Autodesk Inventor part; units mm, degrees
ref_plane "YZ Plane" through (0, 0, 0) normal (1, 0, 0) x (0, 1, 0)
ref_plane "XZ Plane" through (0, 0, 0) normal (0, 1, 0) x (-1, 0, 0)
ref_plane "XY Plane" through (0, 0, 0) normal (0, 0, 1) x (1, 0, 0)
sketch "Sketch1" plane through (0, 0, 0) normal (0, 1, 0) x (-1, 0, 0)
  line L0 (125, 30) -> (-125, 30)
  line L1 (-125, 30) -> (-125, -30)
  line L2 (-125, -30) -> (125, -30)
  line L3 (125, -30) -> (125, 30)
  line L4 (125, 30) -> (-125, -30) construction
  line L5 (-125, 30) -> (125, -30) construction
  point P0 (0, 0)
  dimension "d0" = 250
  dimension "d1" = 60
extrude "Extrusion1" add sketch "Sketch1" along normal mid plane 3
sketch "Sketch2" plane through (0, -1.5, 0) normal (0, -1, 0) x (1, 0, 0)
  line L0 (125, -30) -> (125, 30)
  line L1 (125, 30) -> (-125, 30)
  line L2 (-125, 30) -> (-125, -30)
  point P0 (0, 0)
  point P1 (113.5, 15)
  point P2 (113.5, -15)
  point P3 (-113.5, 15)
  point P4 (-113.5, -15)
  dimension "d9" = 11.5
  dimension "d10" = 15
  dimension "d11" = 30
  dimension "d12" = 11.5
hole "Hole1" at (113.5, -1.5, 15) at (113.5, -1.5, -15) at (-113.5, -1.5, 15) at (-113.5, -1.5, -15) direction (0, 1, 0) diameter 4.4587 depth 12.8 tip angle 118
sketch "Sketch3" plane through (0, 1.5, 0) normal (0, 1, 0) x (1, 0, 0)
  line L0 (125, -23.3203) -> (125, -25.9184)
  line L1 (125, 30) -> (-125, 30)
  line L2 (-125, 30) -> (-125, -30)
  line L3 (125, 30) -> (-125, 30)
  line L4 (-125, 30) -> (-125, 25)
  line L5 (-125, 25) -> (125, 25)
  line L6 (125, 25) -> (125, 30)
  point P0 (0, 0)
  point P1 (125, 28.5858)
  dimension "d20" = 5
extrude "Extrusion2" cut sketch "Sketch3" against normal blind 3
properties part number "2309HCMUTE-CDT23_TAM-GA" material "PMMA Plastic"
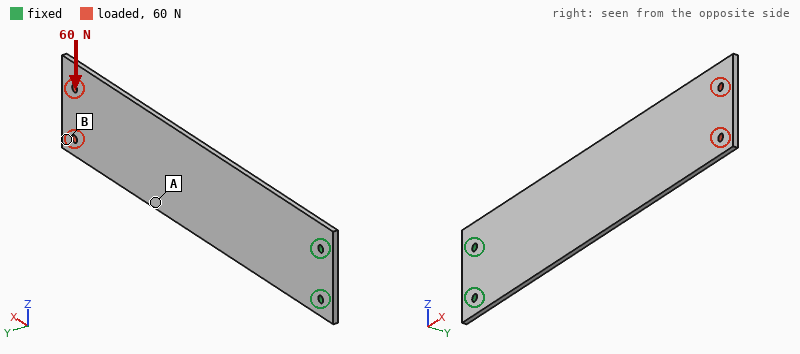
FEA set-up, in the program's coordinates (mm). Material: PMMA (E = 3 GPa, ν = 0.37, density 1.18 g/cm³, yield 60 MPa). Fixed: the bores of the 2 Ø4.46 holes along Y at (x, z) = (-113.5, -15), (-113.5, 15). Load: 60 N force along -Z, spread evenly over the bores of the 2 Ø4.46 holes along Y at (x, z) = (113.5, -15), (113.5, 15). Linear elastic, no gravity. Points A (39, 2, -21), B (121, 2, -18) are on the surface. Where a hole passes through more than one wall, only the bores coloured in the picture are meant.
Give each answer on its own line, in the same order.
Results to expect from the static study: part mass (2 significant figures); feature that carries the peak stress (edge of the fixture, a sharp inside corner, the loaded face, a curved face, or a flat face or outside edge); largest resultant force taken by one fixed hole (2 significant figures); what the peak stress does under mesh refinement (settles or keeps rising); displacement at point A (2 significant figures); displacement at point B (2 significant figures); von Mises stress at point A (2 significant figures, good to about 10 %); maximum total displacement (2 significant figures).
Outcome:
48 g
edge of the fixture
430 N
keeps rising
1.3 mm
2.4 mm
2.6 MPa
2.4 mm
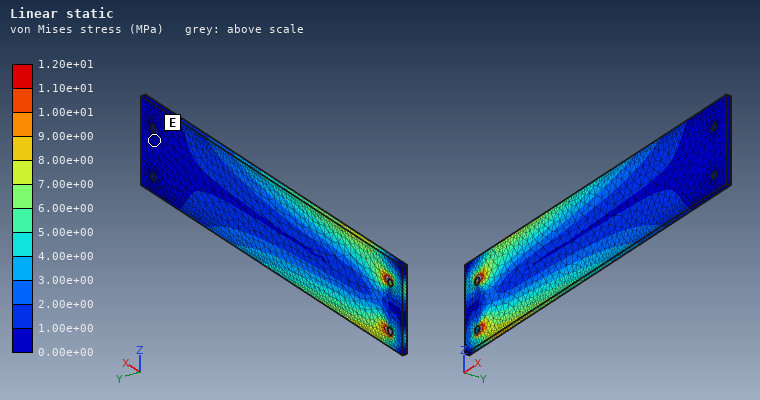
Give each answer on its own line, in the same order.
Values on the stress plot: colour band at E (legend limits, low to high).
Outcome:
0.00e+00 to 1.00e+00 MPa
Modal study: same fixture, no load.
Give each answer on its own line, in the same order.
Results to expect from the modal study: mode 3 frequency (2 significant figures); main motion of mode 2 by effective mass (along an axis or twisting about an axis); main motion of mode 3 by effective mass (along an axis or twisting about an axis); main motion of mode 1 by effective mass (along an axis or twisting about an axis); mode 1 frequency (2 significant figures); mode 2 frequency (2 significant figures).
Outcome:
110 Hz
along Y
twisting about X
along Y
14 Hz
86 Hz
